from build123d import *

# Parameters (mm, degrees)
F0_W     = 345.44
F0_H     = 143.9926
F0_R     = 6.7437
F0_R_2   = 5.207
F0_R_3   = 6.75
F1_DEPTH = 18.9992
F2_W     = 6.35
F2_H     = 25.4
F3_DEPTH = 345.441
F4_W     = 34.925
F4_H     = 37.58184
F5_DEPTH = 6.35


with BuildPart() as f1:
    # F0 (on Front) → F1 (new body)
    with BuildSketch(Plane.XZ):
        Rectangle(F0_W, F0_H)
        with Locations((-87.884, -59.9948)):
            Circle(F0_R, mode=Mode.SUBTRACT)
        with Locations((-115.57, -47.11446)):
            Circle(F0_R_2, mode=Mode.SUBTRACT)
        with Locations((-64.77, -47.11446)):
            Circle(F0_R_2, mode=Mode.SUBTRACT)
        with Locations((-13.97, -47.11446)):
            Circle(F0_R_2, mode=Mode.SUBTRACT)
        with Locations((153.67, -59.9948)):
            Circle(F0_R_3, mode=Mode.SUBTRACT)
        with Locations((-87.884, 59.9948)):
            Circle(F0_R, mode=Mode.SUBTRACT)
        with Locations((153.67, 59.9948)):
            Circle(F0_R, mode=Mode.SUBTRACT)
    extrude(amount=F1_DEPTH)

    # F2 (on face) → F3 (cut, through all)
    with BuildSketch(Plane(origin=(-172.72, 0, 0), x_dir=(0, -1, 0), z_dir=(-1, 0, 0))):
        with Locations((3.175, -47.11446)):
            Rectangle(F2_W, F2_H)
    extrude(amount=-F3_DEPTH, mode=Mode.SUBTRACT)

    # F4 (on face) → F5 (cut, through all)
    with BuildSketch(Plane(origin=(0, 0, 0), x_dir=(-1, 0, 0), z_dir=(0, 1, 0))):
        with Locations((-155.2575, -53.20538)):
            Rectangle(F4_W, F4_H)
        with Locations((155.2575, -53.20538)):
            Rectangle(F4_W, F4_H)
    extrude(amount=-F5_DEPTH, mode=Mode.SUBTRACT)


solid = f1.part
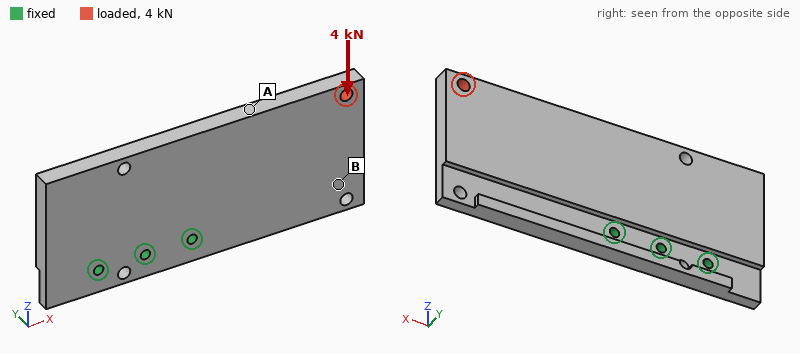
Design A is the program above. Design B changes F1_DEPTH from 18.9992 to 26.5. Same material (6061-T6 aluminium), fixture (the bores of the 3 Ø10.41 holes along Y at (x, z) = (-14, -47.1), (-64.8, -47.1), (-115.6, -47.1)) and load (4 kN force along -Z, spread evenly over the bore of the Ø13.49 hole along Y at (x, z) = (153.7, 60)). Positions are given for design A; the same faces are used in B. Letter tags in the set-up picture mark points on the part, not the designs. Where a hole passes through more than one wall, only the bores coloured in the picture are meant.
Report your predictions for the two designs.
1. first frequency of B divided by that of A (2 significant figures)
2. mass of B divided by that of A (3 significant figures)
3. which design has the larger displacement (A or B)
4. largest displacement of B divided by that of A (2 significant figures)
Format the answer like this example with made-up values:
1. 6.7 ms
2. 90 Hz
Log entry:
1. 1.4
2. 1.42
3. A
4. 0.57
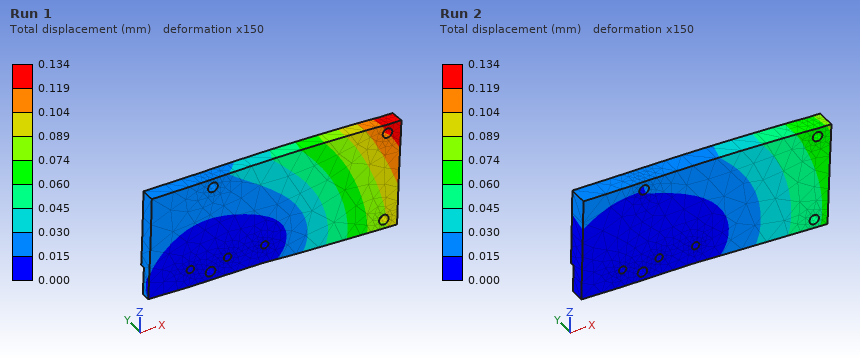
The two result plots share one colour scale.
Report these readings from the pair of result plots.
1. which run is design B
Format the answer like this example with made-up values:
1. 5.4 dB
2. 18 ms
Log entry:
1. Run 2
